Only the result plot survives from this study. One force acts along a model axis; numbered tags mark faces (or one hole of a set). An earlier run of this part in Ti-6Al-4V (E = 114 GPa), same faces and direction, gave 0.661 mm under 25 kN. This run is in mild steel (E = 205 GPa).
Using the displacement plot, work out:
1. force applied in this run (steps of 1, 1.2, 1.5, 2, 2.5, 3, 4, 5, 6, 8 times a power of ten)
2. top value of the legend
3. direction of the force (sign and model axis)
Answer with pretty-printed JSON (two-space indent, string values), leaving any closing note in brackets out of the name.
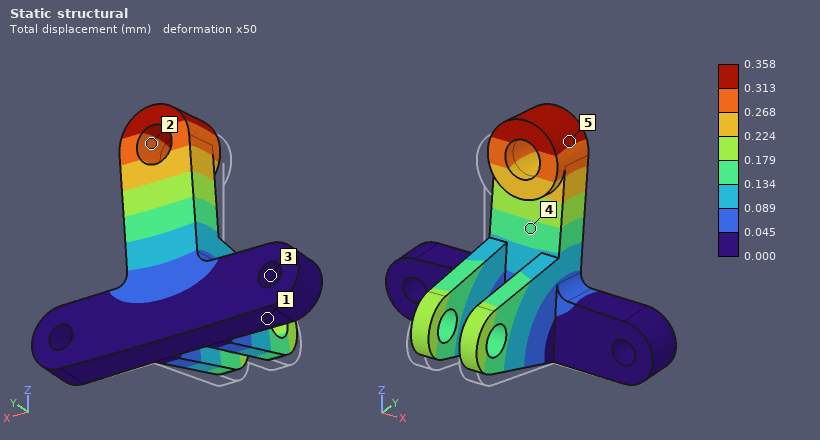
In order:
{
  "force applied in this run": "25 kN",
  "top value of the legend": "0.358 mm",
  "direction of the force": "+Y"
}
